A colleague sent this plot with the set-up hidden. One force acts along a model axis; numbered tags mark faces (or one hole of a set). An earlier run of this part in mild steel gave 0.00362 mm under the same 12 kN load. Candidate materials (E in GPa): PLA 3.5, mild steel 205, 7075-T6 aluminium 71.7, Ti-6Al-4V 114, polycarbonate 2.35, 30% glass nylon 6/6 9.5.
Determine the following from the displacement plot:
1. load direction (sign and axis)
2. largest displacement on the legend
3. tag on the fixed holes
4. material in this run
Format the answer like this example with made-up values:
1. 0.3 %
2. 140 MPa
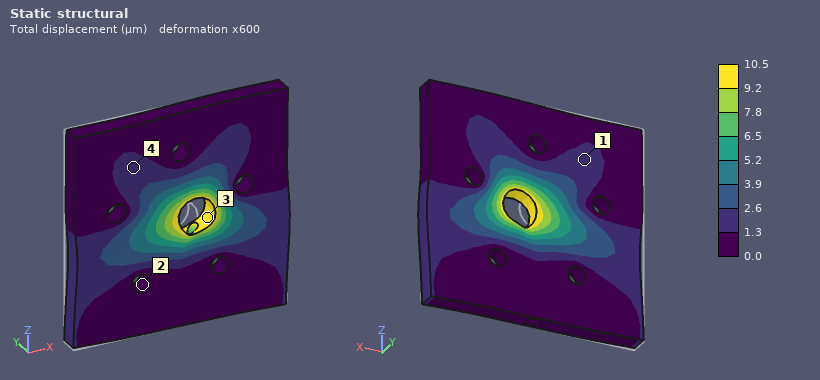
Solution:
1. +X
2. 10.5 µm
3. 2
4. 7075-T6 aluminium
